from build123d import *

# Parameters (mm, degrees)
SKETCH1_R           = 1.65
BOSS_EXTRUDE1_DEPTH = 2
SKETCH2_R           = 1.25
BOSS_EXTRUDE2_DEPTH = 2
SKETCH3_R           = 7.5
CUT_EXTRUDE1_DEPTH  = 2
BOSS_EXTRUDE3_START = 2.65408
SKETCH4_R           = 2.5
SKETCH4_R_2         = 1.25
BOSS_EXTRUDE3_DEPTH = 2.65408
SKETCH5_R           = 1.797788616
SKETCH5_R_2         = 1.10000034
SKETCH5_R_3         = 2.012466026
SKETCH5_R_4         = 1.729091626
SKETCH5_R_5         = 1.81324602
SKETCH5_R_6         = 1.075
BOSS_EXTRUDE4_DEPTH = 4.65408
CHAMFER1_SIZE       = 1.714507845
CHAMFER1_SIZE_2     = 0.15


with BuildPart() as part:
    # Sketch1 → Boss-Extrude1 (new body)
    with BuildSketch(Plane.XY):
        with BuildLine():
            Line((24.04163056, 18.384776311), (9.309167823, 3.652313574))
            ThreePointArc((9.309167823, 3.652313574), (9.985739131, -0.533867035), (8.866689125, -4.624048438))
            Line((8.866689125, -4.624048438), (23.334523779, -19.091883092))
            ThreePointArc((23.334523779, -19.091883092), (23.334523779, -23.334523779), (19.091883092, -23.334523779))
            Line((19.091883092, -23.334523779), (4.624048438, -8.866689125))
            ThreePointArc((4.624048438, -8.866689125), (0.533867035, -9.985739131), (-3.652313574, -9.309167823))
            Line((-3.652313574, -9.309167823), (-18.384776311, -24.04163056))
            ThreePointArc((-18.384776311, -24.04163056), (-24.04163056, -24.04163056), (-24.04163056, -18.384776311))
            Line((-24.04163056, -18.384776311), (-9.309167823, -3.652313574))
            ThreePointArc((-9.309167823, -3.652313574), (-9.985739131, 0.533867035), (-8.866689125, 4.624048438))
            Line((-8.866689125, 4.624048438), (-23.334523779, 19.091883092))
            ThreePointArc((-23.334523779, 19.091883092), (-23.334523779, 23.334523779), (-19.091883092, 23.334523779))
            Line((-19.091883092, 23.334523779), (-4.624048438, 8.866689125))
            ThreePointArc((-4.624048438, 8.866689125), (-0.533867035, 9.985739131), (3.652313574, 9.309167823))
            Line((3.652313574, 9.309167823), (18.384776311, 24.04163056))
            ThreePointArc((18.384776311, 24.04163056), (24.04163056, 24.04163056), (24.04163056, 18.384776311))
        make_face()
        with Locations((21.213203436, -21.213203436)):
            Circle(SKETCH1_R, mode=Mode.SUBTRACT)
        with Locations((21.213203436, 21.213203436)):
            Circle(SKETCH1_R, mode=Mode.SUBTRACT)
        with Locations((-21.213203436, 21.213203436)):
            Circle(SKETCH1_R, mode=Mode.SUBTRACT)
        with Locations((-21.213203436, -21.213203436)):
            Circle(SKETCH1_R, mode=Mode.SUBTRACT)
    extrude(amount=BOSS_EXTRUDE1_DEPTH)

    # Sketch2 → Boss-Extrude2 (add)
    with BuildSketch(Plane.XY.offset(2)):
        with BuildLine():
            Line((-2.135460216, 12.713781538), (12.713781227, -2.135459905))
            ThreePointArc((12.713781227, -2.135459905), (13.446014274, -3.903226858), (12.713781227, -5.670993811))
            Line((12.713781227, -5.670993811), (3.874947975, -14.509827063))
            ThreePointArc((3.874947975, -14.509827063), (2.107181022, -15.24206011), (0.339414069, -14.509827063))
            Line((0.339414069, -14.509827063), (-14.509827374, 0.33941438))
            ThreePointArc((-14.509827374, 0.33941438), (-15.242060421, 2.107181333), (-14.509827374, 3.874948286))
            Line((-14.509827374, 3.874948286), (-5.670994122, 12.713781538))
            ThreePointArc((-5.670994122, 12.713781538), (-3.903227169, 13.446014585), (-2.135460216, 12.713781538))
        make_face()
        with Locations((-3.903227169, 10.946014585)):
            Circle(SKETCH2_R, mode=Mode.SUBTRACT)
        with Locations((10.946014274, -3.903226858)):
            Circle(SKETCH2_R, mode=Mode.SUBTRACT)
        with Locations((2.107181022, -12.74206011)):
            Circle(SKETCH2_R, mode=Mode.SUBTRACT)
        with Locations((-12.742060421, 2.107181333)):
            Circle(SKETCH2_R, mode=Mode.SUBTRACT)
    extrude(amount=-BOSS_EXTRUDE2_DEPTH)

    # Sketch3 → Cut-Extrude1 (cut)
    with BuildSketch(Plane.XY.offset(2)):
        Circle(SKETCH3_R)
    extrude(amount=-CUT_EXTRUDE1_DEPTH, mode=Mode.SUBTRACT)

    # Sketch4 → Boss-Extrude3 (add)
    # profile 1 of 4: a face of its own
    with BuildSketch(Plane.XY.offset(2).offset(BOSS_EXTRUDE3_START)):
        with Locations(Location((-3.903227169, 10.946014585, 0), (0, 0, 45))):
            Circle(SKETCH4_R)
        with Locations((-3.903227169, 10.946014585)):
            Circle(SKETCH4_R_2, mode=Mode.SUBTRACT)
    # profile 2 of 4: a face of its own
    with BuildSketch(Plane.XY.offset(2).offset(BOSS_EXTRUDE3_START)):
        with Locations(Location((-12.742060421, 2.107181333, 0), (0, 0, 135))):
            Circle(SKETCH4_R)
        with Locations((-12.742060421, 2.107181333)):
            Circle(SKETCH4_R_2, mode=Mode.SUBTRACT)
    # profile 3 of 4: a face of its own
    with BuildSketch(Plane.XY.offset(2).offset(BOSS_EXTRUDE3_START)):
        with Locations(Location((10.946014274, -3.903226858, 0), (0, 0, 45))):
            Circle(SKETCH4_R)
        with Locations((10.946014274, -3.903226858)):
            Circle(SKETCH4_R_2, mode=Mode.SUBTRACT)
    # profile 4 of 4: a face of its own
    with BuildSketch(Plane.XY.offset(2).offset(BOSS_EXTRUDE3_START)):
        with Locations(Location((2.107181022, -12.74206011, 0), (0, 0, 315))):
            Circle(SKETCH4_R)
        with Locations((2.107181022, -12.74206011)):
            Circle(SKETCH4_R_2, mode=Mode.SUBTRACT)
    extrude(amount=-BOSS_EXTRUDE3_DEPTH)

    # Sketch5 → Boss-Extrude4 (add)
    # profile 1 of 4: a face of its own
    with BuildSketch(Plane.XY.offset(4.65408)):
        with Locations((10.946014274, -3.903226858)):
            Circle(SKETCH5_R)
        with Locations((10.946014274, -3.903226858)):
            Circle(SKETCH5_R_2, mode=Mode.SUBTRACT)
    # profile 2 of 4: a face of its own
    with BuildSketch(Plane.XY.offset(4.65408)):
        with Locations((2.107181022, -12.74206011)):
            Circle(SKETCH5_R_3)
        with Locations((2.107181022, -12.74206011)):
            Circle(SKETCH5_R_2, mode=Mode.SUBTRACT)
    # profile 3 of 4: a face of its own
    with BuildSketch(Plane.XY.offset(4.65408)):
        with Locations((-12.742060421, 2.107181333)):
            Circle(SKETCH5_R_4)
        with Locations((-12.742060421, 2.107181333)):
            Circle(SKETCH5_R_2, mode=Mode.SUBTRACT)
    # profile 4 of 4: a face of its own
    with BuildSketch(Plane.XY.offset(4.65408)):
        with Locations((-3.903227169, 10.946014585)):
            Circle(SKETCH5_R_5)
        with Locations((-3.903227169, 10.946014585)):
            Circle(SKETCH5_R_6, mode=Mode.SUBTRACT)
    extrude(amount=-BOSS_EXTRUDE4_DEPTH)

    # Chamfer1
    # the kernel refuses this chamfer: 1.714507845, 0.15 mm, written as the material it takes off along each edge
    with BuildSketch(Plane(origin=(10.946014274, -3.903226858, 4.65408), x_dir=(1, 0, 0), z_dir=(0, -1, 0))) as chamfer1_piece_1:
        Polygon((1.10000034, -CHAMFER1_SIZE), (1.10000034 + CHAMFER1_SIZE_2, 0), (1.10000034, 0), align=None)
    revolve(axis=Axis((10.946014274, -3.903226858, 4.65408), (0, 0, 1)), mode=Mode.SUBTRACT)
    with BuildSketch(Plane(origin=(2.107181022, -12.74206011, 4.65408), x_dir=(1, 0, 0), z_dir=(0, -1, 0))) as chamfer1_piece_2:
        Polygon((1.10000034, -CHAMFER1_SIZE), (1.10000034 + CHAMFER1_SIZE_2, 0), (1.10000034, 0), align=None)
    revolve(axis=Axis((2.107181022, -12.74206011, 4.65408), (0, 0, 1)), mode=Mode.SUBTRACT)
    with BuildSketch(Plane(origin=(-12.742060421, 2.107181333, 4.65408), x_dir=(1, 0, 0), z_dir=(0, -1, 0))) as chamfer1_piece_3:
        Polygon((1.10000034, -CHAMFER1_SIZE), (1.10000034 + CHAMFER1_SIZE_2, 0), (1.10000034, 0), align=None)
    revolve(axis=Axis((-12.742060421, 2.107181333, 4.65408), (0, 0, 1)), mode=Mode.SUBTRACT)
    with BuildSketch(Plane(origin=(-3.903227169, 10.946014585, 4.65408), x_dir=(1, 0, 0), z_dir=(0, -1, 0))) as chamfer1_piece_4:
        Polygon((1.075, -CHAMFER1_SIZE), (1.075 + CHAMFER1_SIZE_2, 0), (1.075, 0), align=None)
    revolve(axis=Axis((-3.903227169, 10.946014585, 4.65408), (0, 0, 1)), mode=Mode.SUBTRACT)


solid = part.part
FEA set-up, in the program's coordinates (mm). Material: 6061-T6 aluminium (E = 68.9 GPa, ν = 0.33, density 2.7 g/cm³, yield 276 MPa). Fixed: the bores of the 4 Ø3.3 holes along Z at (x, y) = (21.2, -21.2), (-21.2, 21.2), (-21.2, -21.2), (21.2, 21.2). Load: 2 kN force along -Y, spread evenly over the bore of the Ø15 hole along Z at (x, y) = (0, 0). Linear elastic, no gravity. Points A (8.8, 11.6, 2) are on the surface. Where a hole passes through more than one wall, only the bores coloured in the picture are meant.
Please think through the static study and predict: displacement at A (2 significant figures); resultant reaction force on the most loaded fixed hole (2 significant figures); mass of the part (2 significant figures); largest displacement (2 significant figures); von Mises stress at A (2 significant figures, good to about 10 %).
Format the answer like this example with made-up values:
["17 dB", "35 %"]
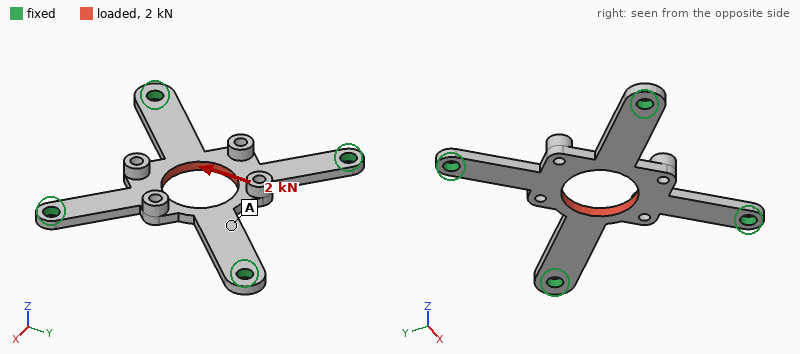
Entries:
["20 µm", "700 N", "5.0 g", "40 µm", "45 MPa"]
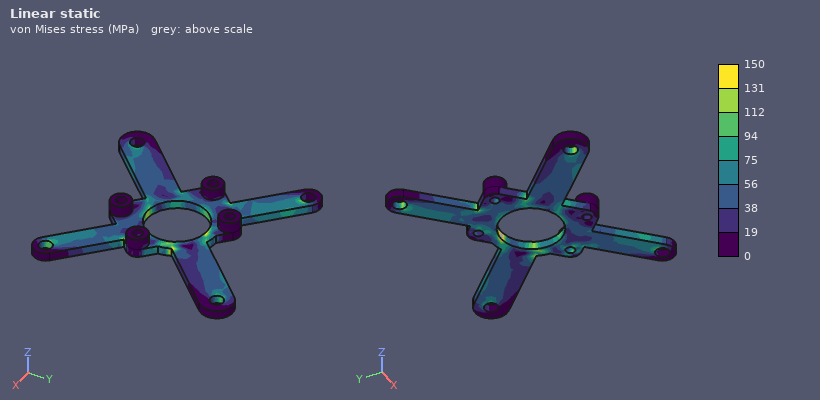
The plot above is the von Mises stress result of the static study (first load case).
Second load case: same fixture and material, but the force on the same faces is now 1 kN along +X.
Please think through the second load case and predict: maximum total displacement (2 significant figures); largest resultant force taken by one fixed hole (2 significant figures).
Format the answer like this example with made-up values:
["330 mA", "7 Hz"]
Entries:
["20 µm", "350 N"]
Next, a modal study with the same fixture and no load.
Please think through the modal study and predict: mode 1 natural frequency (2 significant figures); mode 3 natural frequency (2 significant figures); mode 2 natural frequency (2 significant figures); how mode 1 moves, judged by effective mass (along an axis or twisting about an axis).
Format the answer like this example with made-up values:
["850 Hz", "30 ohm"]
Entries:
["3400 Hz", "6800 Hz", "6700 Hz", "along Z"]
